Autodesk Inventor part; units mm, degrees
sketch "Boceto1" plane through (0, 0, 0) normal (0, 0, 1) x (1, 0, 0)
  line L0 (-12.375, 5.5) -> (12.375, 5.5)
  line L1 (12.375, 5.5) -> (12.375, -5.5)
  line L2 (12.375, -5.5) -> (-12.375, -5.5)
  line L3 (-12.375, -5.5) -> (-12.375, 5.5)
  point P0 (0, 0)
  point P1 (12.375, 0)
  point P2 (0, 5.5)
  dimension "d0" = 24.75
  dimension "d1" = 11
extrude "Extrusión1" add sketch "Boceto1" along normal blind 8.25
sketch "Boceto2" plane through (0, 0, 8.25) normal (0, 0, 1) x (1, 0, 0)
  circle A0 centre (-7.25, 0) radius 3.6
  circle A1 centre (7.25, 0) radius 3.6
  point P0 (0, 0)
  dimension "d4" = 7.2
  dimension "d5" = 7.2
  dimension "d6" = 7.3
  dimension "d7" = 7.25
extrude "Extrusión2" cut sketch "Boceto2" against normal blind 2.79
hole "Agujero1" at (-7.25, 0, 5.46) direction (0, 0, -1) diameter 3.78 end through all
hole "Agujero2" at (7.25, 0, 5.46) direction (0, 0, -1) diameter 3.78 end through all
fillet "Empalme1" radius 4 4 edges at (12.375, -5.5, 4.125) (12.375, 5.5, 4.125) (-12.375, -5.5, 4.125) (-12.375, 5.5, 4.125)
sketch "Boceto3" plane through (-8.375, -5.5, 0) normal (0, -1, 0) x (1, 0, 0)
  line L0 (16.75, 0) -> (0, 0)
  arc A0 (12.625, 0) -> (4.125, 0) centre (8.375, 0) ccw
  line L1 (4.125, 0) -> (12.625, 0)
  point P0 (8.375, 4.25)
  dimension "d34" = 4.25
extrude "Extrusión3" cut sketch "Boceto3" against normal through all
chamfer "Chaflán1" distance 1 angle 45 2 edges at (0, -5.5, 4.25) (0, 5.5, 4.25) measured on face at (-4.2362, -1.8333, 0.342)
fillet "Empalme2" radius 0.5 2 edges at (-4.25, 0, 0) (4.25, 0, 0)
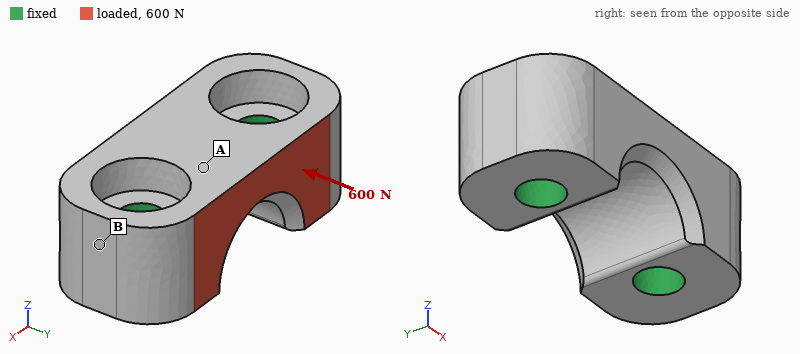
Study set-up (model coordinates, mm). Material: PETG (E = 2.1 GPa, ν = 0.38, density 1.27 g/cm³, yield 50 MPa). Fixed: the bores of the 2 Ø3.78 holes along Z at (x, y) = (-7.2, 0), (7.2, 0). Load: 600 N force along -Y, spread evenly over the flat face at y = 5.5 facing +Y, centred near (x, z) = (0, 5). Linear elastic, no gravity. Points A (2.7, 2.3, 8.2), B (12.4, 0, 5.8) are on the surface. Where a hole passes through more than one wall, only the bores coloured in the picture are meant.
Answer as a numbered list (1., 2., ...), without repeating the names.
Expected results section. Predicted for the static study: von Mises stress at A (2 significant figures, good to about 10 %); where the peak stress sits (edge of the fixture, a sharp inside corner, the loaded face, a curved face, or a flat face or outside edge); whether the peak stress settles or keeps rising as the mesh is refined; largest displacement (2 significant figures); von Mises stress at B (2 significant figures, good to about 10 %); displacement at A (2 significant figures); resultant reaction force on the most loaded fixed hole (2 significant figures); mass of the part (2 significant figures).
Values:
1. 9.9 MPa
2. edge of the fixture
3. keeps rising
4. 91 µm
5. 4.0 MPa
6. 65 µm
7. 300 N
8. 1.8 g
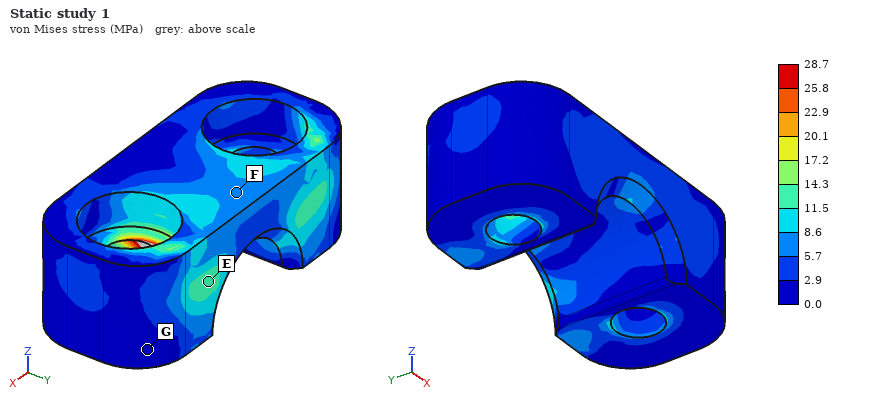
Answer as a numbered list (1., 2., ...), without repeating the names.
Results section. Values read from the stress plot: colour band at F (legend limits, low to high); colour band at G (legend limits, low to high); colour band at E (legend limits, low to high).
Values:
1. 5.7 to 8.6 MPa
2. 0.0 to 2.9 MPa
3. 11.5 to 14.3 MPa
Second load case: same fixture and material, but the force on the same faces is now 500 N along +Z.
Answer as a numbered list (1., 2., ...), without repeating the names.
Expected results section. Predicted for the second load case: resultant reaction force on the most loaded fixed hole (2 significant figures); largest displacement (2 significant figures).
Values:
1. 260 N
2. 0.14 mm
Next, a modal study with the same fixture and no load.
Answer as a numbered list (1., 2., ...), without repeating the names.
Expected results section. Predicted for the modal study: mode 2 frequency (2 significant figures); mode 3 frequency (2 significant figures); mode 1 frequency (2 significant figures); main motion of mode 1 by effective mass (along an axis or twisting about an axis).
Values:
1. 21 kHz
2. 22 kHz
3. 15 kHz
4. along Y
